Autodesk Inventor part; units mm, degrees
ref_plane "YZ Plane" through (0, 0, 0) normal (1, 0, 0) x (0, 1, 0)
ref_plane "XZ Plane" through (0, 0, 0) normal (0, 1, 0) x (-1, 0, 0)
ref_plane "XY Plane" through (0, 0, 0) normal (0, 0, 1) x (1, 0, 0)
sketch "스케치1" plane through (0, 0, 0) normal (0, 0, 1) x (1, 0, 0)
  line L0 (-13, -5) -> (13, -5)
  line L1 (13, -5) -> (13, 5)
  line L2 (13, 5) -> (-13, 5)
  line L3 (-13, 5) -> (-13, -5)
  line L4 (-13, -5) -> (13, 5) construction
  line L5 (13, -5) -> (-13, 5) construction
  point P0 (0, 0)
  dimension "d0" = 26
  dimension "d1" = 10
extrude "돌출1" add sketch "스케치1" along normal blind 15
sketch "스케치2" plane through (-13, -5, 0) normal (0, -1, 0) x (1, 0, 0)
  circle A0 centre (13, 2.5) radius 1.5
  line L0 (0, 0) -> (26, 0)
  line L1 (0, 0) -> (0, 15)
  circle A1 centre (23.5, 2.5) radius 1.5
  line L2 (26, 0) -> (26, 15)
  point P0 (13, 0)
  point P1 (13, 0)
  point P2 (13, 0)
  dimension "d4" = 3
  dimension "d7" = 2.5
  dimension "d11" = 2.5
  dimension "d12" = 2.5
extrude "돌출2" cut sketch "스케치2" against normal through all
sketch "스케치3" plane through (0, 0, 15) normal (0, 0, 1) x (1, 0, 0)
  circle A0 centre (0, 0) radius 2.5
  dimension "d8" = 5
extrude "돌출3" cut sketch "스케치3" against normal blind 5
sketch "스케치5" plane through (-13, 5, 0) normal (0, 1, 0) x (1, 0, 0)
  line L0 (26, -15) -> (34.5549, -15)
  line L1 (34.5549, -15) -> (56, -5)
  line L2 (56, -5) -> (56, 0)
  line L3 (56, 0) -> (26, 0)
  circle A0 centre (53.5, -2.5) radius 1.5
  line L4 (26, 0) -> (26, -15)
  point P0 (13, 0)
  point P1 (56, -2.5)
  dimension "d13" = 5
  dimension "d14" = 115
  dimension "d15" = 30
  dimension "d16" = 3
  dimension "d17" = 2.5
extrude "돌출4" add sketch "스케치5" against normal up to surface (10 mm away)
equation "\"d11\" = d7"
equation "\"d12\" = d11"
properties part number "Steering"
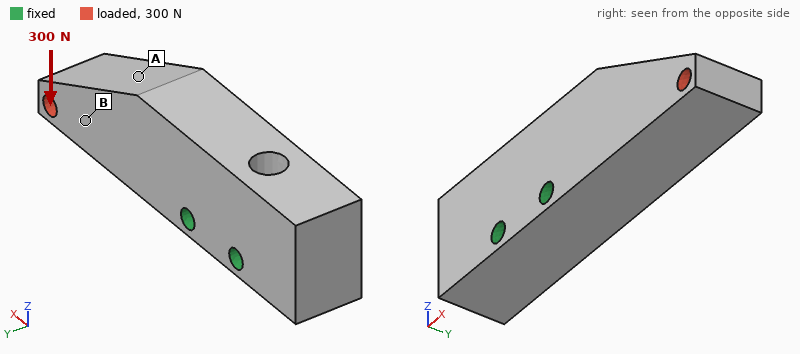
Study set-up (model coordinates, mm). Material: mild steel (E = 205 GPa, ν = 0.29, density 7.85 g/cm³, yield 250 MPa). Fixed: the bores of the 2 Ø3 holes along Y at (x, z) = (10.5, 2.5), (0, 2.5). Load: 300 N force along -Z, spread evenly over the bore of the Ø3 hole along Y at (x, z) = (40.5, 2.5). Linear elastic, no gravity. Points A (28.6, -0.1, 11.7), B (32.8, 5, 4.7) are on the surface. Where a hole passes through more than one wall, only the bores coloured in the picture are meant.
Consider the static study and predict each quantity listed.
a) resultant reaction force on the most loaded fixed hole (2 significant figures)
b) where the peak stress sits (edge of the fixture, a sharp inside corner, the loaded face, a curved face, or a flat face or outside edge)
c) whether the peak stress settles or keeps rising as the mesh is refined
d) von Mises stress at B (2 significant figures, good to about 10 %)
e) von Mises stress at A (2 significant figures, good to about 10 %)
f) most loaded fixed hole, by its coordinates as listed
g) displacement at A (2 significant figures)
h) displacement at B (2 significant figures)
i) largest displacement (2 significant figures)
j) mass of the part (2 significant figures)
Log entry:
990 N
edge of the fixture
keeps rising
5.1 MPa
18 MPa
(10.5, 2.5)
4.9 µm
6.1 µm
12 µm
55 g
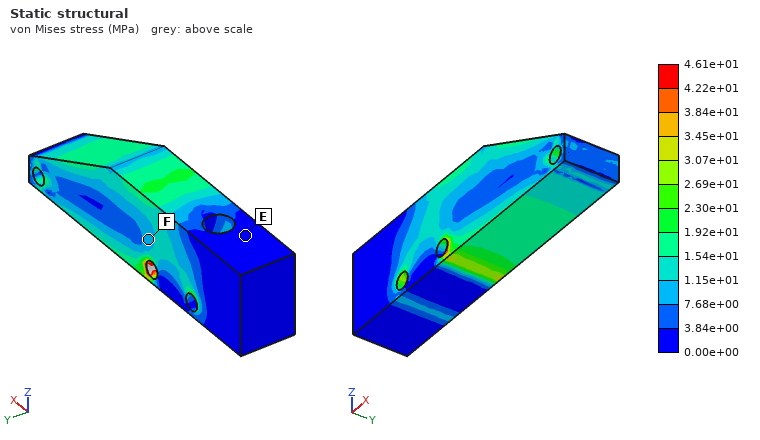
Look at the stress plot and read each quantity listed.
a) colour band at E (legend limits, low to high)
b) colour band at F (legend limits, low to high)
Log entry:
0.00e+00 to 3.84e+00 MPa
7.68e+00 to 1.15e+01 MPa
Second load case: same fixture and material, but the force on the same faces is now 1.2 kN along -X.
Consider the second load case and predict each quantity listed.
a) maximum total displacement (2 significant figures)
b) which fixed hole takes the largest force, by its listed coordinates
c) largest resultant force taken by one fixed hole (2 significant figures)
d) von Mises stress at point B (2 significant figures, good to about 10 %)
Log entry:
7.5 µm
(10.5, 2.5)
1.1 kN
13 MPa
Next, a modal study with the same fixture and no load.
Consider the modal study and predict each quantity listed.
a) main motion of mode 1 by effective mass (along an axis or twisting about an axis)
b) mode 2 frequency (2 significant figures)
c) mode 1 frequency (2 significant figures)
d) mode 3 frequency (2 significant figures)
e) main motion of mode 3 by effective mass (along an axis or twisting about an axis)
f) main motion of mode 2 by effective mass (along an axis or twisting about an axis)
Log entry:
along Y
11 kHz
9100 Hz
24 kHz
along Y
along Z
